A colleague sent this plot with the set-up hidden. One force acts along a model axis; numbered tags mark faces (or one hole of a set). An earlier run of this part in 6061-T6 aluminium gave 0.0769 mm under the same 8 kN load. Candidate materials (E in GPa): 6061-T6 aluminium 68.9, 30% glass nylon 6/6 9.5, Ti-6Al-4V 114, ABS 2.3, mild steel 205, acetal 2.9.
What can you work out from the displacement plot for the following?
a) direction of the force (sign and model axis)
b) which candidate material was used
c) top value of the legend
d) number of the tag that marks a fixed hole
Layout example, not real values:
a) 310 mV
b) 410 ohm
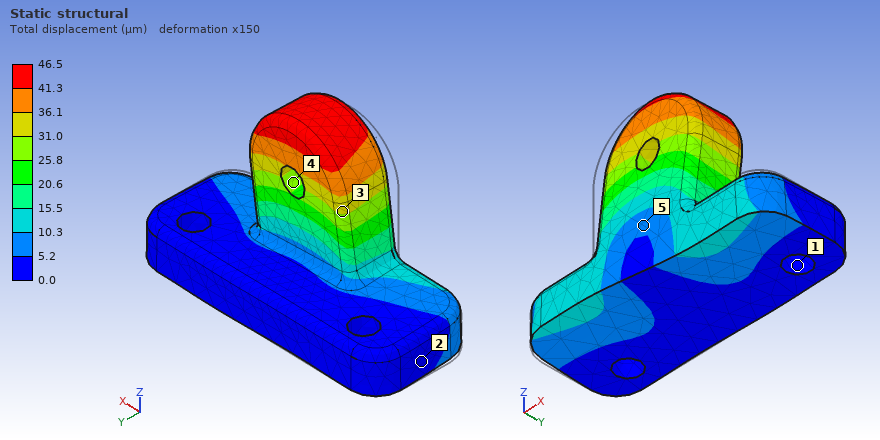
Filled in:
a) +X
b) Ti-6Al-4V
c) 46.5 µm
d) 1
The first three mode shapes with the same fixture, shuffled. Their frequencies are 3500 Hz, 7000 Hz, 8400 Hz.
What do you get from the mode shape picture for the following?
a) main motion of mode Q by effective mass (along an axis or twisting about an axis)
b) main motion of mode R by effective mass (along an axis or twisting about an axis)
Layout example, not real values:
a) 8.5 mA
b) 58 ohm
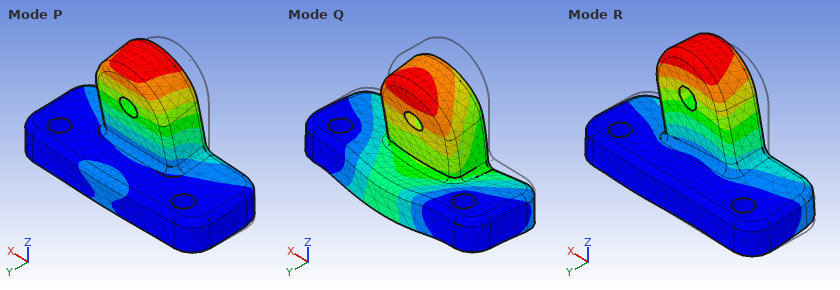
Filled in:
a) along Z
b) along X
